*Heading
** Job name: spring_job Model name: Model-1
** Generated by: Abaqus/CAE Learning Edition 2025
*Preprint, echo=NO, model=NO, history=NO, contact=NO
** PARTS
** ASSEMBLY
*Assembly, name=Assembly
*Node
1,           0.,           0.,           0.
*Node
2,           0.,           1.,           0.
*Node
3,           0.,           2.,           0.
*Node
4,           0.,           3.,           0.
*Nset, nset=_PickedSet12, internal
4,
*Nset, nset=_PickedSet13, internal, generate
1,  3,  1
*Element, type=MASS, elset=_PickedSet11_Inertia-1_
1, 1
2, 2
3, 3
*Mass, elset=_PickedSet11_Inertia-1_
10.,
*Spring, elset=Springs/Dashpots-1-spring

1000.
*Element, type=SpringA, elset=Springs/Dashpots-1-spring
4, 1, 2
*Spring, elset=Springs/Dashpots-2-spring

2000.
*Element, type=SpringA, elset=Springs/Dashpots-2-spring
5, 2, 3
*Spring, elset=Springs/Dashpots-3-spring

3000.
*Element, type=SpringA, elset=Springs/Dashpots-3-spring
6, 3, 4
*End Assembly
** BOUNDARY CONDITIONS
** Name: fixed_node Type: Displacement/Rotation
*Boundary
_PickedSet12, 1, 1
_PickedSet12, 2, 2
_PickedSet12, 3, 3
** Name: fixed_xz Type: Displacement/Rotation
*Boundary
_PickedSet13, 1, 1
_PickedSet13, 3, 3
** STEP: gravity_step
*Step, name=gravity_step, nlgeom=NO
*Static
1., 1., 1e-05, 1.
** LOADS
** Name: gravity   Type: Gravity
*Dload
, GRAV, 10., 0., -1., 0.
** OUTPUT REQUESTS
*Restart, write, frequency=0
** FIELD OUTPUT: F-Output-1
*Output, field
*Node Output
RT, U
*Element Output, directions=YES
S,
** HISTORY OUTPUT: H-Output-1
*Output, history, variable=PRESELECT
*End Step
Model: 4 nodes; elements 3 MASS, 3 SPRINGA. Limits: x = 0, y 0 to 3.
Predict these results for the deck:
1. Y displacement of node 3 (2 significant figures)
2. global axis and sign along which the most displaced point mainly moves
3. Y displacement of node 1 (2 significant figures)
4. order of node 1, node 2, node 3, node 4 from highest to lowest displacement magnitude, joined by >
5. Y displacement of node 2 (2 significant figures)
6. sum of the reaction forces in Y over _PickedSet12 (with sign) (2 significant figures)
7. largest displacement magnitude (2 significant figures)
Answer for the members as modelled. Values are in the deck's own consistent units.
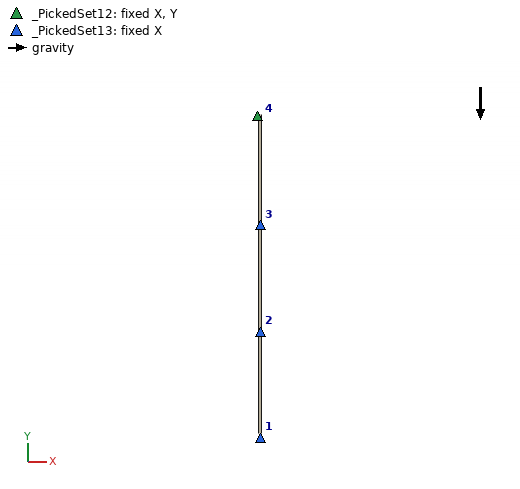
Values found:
-0.10
-Y
-0.30
node 1 > node 2 > node 3 > node 4
-0.20
300
0.30
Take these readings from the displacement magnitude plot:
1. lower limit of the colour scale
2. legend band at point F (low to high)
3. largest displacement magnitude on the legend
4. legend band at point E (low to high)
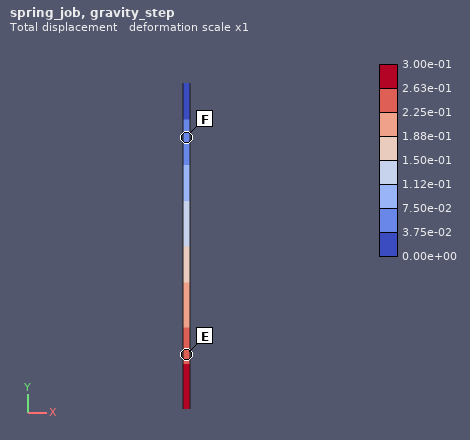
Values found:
0.00e+00
3.75e-02 to 7.50e-02
3.00e-01
2.25e-01 to 2.63e-01
